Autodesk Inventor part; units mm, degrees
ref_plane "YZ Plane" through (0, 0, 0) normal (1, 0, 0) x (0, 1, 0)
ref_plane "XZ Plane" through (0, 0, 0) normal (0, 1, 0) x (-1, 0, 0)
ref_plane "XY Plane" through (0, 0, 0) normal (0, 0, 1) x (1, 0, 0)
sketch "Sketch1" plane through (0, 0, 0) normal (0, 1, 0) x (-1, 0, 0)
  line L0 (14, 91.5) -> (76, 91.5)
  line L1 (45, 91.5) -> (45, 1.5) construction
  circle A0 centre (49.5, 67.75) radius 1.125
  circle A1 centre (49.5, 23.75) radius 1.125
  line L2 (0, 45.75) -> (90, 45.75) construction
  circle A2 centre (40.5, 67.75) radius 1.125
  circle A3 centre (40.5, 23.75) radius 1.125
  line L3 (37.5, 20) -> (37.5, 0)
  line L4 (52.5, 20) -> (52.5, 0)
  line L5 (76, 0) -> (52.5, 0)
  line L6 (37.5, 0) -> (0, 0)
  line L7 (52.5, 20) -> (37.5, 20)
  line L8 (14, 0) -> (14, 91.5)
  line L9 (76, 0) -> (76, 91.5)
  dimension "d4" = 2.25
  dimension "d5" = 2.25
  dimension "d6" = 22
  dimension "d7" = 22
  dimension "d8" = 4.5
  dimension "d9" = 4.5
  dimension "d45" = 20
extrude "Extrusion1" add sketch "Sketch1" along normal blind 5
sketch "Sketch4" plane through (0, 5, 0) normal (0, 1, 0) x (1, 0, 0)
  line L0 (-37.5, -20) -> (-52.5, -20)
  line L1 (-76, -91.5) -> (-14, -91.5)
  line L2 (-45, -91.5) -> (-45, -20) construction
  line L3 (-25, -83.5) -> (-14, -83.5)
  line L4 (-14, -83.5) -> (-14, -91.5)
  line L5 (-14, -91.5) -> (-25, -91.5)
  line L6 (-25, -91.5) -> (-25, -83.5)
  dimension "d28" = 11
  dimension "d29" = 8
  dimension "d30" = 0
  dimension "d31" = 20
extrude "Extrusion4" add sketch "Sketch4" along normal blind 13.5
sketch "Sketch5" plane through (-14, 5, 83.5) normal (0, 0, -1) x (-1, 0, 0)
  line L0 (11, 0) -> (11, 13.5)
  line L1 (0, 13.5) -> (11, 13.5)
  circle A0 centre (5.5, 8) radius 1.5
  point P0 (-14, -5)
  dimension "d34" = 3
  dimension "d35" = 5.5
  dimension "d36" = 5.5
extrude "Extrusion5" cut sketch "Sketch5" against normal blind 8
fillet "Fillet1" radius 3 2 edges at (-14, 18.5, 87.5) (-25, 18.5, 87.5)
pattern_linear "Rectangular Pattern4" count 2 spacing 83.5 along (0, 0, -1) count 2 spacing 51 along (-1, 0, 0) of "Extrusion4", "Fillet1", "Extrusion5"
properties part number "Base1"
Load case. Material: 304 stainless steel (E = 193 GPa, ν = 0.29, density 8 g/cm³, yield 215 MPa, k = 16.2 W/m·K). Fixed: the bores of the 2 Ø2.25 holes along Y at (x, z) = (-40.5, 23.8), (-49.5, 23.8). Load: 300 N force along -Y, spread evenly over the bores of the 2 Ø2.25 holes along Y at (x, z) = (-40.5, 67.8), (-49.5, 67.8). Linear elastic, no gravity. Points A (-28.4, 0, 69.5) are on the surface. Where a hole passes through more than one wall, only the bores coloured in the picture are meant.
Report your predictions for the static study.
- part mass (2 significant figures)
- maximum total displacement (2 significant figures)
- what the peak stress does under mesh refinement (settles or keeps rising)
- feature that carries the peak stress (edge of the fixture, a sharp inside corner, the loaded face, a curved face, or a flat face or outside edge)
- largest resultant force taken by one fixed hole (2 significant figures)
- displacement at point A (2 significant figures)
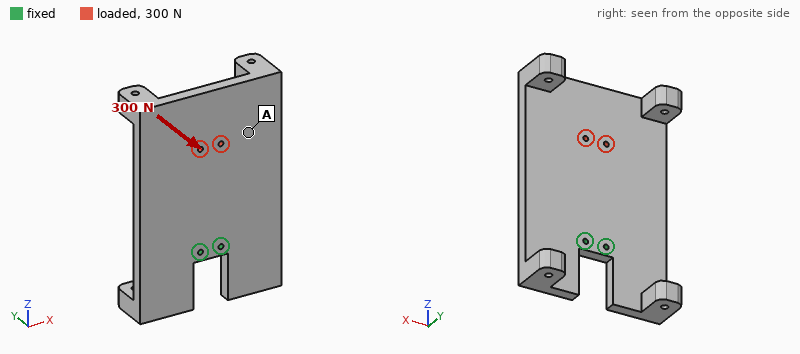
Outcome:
250 g
0.19 mm
keeps rising
edge of the fixture
150 N
0.12 mm
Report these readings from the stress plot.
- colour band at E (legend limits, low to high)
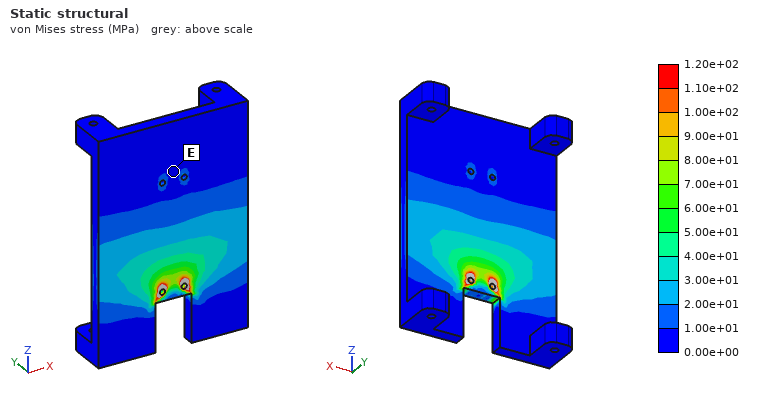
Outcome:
0.00e+00 to 1.00e+01 MPa
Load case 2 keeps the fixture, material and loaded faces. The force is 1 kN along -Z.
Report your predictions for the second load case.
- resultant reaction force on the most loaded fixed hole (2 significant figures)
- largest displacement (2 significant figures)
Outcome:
500 N
1.8 µm
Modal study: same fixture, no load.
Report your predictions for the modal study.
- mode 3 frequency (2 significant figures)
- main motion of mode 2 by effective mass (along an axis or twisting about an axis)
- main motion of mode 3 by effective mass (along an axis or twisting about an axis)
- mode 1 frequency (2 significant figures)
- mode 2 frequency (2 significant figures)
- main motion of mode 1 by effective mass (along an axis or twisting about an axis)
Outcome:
1600 Hz
twisting about Z
along X
600 Hz
1300 Hz
along Y
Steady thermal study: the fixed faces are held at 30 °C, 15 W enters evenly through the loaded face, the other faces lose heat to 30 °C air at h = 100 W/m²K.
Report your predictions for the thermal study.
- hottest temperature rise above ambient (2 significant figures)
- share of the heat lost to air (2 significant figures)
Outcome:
67 K
94 %
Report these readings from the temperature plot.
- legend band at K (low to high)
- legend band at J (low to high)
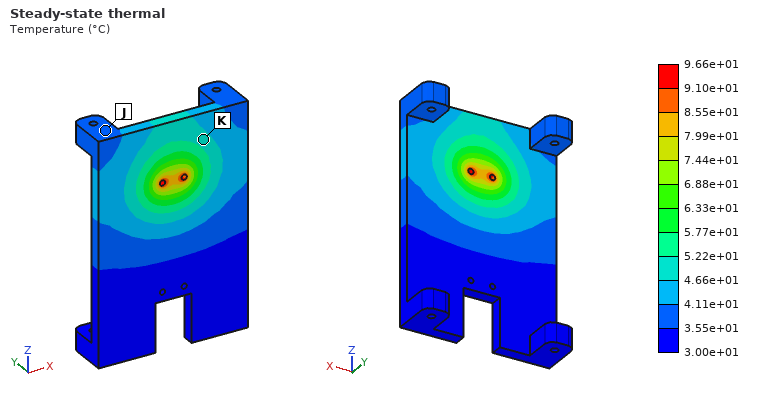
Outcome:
4.66e+01 to 5.22e+01 °C
3.55e+01 to 4.11e+01 °C
